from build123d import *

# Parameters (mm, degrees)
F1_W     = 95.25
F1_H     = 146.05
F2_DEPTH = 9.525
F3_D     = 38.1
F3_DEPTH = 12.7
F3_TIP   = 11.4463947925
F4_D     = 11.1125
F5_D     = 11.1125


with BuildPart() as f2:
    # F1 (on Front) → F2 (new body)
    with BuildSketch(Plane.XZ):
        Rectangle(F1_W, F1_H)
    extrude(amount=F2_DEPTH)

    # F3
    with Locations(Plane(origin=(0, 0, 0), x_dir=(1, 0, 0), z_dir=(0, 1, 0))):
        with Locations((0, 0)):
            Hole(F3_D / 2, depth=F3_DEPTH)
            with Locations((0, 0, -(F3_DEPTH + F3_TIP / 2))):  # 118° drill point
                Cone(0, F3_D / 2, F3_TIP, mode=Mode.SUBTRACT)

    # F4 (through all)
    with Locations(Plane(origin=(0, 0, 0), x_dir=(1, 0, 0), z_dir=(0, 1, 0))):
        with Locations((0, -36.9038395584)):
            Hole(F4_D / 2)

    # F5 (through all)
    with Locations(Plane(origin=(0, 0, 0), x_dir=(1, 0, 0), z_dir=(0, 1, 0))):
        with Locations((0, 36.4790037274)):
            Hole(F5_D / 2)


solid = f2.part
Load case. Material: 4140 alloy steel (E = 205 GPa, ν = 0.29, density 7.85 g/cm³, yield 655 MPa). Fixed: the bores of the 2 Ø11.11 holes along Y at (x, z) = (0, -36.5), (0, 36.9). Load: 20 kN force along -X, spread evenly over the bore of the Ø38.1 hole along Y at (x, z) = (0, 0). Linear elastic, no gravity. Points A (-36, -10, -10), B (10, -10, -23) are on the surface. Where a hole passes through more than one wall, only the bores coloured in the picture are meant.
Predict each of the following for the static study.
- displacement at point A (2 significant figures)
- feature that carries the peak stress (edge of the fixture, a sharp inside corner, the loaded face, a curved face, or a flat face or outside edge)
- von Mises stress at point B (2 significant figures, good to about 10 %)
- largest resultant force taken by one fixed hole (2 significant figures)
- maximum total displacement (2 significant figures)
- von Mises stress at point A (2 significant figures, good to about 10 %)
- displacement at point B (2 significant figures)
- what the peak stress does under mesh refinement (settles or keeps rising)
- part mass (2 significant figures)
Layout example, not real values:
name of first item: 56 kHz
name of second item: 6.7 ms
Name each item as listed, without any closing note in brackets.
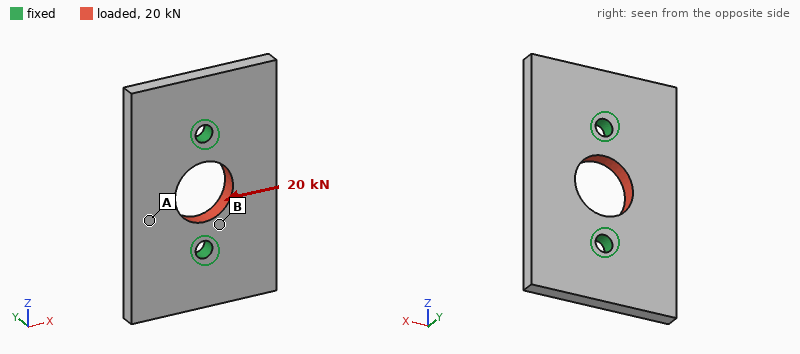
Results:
displacement at point A: 5.0 µm
feature that carries the peak stress: edge of the fixture
von Mises stress at point B: 30 MPa
largest resultant force taken by one fixed hole: 10 kN
maximum total displacement: 6.6 µm
von Mises stress at point A: 16 MPa
displacement at point B: 3.2 µm
what the peak stress does under mesh refinement: keeps rising
part mass: 940 g
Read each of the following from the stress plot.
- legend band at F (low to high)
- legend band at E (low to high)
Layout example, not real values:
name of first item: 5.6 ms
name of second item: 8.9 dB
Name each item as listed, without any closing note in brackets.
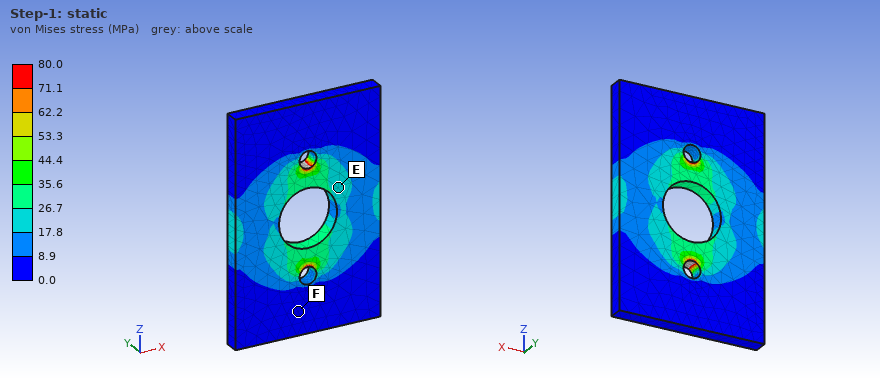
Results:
legend band at F: 0.0 to 8.9 MPa
legend band at E: 17.8 to 26.7 MPa
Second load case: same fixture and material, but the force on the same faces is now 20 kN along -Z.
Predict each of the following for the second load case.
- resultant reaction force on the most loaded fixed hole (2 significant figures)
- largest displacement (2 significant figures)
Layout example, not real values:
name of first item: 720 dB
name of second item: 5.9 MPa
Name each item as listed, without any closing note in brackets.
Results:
resultant reaction force on the most loaded fixed hole: 10 kN
largest displacement: 5.0 µm
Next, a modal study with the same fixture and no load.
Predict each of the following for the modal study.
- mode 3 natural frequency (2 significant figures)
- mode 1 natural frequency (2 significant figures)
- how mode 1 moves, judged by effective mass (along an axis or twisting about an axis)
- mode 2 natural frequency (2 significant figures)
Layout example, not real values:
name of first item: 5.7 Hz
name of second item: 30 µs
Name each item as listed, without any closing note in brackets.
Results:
mode 3 natural frequency: 3300 Hz
mode 1 natural frequency: 2700 Hz
how mode 1 moves, judged by effective mass: twisting about Z
mode 2 natural frequency: 3200 Hz
